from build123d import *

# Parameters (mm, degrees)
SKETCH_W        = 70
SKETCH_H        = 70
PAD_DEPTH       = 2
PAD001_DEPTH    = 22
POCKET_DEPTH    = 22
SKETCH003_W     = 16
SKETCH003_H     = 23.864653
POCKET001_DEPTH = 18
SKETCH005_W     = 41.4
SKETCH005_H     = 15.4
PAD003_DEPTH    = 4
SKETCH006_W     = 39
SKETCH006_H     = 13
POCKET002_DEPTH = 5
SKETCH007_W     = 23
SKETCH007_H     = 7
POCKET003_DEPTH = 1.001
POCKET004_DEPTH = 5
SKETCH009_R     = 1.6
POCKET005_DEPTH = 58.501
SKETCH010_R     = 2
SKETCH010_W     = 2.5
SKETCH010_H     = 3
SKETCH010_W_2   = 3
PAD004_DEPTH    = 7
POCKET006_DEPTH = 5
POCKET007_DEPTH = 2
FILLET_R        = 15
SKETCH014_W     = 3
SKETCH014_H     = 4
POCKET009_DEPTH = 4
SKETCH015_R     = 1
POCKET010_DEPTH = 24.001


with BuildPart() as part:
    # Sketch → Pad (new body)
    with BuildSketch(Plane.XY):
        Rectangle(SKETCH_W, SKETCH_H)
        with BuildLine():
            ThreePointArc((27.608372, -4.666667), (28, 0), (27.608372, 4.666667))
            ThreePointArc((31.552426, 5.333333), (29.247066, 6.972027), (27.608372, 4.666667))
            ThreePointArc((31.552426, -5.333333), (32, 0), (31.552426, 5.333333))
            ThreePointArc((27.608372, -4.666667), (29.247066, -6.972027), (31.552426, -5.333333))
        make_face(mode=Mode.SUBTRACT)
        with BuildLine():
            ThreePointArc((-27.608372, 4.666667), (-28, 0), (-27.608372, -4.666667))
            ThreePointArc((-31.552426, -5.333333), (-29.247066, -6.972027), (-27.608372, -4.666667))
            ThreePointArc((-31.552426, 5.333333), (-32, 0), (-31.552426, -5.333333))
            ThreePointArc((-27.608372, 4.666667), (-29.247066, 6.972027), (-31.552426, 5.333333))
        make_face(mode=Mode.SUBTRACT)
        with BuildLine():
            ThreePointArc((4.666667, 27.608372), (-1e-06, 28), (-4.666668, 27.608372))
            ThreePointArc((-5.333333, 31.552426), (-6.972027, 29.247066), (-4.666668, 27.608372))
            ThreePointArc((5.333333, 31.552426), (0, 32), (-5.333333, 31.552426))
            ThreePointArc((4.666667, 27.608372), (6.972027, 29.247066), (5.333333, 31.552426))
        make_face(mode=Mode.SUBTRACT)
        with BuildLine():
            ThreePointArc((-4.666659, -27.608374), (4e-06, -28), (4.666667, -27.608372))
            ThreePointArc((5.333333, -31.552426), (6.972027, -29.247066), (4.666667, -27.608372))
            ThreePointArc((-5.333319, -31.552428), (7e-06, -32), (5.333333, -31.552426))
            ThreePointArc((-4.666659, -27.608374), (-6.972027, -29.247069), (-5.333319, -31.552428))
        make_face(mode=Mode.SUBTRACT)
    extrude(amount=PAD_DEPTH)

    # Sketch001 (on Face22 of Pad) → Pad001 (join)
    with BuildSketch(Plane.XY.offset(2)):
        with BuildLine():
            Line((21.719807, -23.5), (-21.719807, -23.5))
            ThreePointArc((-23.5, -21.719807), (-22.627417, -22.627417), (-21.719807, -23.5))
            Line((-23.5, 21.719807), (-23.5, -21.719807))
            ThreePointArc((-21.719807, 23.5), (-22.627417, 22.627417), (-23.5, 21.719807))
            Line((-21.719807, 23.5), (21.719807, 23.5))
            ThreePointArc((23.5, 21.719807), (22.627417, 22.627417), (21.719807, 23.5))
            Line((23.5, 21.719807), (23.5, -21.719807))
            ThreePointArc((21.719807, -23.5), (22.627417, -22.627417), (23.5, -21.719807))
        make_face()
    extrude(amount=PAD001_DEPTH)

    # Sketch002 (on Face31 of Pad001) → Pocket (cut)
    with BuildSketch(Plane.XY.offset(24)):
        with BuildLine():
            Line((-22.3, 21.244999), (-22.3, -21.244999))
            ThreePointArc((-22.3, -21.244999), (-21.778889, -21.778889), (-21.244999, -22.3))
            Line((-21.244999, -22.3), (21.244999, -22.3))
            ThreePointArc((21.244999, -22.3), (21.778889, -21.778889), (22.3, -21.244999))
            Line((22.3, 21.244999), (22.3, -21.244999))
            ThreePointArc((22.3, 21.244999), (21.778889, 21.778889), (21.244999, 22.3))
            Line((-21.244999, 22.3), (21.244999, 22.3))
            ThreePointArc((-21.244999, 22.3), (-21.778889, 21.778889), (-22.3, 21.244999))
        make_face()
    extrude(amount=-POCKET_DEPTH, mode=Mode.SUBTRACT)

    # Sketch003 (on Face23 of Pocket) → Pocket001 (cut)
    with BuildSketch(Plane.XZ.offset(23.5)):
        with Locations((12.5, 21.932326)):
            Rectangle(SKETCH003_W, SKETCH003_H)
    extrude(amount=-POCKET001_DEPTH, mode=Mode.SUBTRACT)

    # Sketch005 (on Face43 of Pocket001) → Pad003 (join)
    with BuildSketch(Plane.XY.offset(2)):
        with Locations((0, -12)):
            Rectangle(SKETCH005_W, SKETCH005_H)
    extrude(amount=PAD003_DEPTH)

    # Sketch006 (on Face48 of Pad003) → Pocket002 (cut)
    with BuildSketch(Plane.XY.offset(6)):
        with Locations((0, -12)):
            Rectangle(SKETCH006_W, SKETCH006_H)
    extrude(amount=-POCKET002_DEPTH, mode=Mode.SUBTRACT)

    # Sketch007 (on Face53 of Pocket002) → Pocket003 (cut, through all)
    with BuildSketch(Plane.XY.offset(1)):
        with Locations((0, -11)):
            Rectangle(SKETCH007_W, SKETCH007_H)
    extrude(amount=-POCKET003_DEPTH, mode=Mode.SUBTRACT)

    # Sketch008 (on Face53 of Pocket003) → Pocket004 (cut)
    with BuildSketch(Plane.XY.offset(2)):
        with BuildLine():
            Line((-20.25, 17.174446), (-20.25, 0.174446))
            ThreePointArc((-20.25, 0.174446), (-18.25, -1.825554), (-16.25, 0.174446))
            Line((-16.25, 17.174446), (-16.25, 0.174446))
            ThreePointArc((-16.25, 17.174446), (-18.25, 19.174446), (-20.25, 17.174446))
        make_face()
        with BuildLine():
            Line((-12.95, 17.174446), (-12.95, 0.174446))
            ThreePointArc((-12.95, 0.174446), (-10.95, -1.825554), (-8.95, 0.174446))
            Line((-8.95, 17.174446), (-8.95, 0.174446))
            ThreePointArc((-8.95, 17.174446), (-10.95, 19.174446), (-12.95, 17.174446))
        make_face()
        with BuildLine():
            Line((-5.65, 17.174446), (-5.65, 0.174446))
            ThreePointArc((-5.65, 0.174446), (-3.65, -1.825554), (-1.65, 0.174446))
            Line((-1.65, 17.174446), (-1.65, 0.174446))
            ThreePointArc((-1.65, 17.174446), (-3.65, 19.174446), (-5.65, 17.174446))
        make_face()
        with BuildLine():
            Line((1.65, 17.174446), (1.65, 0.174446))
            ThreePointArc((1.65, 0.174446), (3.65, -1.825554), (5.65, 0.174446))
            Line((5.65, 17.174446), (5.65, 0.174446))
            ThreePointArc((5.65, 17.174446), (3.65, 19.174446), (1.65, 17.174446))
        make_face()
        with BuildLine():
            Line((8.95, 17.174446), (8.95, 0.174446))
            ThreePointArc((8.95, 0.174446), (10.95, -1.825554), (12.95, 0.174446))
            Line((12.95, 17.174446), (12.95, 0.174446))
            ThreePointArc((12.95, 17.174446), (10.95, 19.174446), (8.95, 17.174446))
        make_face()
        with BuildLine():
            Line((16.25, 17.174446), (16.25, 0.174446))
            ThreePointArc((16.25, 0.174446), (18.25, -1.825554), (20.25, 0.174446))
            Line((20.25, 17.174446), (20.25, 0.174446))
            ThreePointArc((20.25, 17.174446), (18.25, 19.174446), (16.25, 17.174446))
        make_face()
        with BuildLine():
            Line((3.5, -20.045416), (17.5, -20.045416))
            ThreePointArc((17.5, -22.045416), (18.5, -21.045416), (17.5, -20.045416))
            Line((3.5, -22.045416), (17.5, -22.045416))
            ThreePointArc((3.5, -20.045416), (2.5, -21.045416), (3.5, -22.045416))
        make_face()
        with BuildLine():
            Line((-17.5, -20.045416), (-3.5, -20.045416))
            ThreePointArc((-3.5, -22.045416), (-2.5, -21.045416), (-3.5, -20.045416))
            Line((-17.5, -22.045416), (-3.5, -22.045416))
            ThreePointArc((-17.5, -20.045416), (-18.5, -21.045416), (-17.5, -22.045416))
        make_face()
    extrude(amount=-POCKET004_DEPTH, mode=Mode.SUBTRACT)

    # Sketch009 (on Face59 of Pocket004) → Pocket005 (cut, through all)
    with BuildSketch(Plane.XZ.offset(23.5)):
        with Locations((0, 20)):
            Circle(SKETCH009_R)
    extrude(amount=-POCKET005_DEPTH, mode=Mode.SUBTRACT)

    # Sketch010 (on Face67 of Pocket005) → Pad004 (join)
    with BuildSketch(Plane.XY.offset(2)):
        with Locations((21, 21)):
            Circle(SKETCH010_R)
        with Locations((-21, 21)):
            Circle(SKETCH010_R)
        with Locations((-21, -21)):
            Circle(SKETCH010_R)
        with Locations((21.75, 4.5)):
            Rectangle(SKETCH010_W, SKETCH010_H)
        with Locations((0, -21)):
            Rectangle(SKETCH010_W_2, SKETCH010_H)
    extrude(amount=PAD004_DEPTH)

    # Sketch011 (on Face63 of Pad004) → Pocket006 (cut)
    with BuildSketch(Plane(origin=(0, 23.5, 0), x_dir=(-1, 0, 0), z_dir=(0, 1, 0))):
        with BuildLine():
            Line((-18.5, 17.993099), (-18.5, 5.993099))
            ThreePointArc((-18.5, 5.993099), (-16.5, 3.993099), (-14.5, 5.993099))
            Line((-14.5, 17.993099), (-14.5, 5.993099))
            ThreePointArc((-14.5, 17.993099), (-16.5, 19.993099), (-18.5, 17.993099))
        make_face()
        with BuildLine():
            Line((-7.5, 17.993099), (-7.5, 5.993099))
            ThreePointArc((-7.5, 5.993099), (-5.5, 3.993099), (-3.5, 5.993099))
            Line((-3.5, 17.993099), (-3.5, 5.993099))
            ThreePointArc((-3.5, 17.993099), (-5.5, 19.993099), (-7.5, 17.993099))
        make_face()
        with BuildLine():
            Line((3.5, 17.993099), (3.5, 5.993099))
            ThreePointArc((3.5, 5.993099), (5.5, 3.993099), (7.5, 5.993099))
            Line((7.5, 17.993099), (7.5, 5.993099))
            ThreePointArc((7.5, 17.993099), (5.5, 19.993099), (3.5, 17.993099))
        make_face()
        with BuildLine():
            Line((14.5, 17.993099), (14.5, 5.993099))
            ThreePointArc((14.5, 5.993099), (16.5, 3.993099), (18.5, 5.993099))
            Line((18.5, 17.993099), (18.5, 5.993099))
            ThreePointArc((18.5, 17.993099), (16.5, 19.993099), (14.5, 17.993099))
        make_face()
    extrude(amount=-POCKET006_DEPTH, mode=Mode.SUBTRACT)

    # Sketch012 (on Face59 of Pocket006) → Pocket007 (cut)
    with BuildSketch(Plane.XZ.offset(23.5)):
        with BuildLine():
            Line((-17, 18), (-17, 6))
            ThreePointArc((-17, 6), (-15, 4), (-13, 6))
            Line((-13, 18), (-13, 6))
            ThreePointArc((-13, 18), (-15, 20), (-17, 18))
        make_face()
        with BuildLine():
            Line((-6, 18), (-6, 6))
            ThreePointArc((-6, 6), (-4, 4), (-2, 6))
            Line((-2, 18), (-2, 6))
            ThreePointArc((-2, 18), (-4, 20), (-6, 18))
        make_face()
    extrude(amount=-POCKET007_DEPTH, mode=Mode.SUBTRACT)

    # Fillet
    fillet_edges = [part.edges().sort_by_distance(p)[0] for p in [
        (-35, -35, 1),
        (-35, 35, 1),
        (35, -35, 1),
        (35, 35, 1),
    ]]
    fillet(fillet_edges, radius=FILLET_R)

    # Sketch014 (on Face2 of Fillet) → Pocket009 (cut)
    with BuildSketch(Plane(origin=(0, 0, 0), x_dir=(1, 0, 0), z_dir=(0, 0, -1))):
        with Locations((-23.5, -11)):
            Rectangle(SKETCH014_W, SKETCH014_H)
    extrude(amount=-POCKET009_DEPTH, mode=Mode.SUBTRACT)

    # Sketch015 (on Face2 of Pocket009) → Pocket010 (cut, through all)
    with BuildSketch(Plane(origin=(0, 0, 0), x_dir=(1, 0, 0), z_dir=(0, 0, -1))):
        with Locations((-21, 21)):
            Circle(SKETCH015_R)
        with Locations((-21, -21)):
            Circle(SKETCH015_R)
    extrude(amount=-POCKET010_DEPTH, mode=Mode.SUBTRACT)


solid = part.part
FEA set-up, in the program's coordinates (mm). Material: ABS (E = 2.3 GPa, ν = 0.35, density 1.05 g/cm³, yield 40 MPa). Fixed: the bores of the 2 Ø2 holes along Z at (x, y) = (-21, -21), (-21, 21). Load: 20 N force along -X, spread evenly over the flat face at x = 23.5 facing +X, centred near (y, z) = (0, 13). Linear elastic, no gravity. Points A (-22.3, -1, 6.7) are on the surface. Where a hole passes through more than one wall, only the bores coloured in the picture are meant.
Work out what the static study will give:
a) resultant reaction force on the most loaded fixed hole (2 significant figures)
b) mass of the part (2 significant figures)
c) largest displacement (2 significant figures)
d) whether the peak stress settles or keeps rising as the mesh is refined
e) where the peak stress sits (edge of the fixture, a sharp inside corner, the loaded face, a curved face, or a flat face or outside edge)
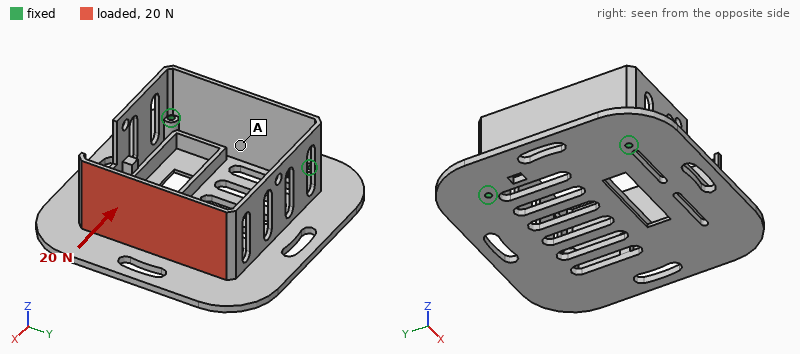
11 N
13 g
1.00 mm
keeps rising
a sharp inside corner
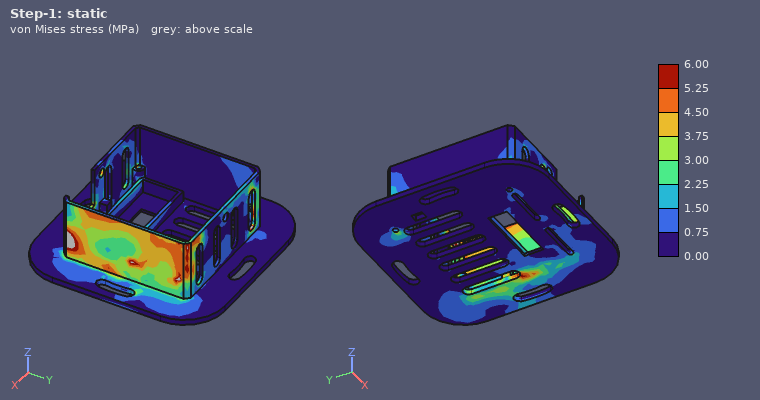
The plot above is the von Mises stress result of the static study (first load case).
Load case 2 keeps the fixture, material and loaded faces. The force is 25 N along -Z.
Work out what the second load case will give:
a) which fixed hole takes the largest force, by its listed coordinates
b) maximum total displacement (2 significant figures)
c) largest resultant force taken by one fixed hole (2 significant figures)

(-21, -21)
1.1 mm
16 N
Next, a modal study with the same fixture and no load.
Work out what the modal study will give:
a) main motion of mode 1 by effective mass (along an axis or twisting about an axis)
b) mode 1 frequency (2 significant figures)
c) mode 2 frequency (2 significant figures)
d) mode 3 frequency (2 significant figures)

along Z
380 Hz
480 Hz
890 Hz
